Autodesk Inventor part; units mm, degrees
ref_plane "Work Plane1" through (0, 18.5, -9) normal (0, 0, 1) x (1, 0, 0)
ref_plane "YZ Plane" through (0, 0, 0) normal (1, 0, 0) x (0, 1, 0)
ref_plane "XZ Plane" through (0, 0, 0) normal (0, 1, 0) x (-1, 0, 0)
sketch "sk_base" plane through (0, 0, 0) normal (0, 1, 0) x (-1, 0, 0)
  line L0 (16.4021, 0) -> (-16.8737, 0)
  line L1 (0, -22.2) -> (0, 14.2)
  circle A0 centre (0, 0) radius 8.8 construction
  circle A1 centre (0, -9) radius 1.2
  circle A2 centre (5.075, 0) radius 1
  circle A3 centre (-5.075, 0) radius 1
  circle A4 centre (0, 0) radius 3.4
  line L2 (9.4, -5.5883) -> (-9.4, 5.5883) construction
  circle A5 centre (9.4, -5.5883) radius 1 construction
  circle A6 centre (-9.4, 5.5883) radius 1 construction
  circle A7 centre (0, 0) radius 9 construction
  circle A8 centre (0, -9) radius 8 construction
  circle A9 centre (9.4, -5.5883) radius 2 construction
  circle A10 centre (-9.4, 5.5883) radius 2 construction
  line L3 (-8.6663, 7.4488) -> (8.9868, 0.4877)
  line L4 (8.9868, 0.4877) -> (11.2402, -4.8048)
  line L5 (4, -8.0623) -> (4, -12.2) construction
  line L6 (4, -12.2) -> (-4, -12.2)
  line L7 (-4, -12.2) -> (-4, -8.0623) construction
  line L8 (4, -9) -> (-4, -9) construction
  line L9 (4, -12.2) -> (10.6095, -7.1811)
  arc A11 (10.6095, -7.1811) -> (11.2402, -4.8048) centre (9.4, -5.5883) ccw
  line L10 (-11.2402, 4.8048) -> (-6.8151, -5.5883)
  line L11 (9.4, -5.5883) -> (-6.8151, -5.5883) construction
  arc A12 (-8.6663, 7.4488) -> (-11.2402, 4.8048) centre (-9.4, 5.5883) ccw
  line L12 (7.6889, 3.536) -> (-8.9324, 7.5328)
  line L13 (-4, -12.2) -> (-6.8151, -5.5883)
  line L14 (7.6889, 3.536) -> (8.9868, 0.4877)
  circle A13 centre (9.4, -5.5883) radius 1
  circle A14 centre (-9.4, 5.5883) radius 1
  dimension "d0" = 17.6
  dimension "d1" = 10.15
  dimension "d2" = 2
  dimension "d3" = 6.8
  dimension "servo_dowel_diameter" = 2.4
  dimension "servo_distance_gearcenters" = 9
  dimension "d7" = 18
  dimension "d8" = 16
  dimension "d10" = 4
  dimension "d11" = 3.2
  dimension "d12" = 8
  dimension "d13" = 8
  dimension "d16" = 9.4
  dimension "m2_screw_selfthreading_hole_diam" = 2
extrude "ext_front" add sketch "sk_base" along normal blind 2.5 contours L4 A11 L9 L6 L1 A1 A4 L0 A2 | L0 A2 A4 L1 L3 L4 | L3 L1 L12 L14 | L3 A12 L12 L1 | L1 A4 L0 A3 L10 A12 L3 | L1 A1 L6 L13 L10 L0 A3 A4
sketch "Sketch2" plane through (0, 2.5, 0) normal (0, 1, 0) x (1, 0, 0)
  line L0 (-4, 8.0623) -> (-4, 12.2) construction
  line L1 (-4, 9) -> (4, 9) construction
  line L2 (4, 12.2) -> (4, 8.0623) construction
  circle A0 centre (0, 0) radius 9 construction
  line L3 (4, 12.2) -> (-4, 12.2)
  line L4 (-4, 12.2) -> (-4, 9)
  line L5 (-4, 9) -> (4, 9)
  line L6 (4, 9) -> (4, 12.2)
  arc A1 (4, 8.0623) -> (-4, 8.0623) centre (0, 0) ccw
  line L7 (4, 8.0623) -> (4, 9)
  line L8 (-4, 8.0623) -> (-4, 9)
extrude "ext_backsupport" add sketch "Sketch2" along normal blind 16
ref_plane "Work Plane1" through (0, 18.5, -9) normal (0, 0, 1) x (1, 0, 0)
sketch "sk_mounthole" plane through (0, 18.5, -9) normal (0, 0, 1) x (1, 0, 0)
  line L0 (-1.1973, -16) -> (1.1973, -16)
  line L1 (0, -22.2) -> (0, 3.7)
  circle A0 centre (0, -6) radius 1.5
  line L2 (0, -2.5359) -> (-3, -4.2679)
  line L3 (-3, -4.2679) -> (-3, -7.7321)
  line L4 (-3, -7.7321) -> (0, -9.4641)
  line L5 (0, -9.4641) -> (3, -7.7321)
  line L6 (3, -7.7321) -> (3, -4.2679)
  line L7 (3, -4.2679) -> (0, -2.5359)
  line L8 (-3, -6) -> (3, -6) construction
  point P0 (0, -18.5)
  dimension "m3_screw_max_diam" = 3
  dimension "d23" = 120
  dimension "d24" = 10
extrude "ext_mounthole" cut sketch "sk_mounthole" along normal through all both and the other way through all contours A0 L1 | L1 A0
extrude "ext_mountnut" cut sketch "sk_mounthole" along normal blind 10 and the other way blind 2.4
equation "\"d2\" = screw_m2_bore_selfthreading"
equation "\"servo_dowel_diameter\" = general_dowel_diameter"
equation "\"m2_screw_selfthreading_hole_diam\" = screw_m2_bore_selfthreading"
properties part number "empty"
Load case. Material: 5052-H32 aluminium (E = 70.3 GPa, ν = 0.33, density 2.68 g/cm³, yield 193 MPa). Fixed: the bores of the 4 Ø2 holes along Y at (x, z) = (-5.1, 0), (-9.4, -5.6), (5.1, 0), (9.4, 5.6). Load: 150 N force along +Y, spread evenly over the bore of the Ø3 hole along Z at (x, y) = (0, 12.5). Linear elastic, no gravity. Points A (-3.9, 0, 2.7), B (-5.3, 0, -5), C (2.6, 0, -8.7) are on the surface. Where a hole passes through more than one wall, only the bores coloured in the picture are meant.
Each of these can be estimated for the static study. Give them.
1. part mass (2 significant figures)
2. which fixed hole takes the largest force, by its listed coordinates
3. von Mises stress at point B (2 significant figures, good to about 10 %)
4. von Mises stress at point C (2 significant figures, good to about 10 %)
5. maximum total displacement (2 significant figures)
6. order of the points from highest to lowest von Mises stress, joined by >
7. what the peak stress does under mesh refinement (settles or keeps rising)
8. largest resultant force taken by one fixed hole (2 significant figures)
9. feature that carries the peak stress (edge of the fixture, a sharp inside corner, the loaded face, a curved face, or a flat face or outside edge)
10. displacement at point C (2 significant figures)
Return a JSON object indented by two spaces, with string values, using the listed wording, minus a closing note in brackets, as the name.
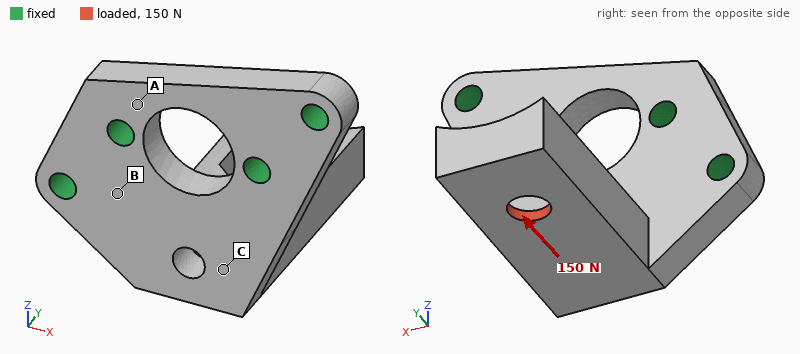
{
  "part mass": "2.6 g",
  "which fixed hole takes the largest force, by its listed coordinates": "(-9.4, -5.6)",
  "von Mises stress at point B": "55 MPa",
  "von Mises stress at point C": "33 MPa",
  "maximum total displacement": "0.12 mm",
  "order of the points from highest to lowest von Mises stress, joined by >": "B > C > A",
  "what the peak stress does under mesh refinement": "keeps rising",
  "largest resultant force taken by one fixed hole": "120 N",
  "feature that carries the peak stress": "edge of the fixture",
  "displacement at point C": "0.028 mm"
}
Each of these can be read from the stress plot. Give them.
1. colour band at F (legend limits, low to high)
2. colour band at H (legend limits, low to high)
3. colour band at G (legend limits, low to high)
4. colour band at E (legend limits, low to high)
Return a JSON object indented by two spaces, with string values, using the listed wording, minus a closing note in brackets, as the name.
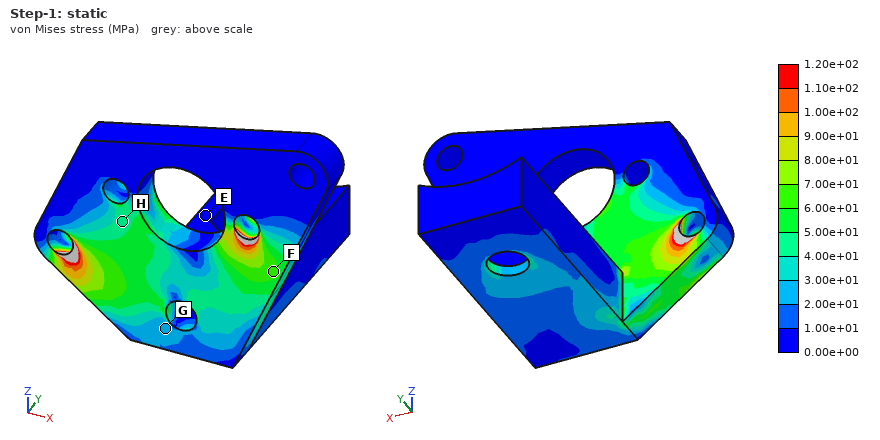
{
  "colour band at F": "6.00e+01 to 7.00e+01 MPa",
  "colour band at H": "4.00e+01 to 5.00e+01 MPa",
  "colour band at G": "2.00e+01 to 3.00e+01 MPa",
  "colour band at E": "0.00e+00 to 1.00e+01 MPa"
}
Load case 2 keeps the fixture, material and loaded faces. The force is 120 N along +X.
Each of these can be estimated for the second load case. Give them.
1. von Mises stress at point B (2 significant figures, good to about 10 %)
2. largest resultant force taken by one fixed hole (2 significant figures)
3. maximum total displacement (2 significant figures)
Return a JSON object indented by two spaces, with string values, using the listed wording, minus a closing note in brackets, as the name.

{
  "von Mises stress at point B": "18 MPa",
  "largest resultant force taken by one fixed hole": "130 N",
  "maximum total displacement": "79 µm"
}
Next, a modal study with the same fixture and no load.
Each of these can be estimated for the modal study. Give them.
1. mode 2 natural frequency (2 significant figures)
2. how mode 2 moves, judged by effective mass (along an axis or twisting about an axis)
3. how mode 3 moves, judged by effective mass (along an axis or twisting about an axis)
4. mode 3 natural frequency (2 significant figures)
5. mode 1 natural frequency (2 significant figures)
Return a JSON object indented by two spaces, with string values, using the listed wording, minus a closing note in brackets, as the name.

{
  "mode 2 natural frequency": "9100 Hz",
  "how mode 2 moves, judged by effective mass": "along X",
  "how mode 3 moves, judged by effective mass": "along Y",
  "mode 3 natural frequency": "17 kHz",
  "mode 1 natural frequency": "5000 Hz"
}
